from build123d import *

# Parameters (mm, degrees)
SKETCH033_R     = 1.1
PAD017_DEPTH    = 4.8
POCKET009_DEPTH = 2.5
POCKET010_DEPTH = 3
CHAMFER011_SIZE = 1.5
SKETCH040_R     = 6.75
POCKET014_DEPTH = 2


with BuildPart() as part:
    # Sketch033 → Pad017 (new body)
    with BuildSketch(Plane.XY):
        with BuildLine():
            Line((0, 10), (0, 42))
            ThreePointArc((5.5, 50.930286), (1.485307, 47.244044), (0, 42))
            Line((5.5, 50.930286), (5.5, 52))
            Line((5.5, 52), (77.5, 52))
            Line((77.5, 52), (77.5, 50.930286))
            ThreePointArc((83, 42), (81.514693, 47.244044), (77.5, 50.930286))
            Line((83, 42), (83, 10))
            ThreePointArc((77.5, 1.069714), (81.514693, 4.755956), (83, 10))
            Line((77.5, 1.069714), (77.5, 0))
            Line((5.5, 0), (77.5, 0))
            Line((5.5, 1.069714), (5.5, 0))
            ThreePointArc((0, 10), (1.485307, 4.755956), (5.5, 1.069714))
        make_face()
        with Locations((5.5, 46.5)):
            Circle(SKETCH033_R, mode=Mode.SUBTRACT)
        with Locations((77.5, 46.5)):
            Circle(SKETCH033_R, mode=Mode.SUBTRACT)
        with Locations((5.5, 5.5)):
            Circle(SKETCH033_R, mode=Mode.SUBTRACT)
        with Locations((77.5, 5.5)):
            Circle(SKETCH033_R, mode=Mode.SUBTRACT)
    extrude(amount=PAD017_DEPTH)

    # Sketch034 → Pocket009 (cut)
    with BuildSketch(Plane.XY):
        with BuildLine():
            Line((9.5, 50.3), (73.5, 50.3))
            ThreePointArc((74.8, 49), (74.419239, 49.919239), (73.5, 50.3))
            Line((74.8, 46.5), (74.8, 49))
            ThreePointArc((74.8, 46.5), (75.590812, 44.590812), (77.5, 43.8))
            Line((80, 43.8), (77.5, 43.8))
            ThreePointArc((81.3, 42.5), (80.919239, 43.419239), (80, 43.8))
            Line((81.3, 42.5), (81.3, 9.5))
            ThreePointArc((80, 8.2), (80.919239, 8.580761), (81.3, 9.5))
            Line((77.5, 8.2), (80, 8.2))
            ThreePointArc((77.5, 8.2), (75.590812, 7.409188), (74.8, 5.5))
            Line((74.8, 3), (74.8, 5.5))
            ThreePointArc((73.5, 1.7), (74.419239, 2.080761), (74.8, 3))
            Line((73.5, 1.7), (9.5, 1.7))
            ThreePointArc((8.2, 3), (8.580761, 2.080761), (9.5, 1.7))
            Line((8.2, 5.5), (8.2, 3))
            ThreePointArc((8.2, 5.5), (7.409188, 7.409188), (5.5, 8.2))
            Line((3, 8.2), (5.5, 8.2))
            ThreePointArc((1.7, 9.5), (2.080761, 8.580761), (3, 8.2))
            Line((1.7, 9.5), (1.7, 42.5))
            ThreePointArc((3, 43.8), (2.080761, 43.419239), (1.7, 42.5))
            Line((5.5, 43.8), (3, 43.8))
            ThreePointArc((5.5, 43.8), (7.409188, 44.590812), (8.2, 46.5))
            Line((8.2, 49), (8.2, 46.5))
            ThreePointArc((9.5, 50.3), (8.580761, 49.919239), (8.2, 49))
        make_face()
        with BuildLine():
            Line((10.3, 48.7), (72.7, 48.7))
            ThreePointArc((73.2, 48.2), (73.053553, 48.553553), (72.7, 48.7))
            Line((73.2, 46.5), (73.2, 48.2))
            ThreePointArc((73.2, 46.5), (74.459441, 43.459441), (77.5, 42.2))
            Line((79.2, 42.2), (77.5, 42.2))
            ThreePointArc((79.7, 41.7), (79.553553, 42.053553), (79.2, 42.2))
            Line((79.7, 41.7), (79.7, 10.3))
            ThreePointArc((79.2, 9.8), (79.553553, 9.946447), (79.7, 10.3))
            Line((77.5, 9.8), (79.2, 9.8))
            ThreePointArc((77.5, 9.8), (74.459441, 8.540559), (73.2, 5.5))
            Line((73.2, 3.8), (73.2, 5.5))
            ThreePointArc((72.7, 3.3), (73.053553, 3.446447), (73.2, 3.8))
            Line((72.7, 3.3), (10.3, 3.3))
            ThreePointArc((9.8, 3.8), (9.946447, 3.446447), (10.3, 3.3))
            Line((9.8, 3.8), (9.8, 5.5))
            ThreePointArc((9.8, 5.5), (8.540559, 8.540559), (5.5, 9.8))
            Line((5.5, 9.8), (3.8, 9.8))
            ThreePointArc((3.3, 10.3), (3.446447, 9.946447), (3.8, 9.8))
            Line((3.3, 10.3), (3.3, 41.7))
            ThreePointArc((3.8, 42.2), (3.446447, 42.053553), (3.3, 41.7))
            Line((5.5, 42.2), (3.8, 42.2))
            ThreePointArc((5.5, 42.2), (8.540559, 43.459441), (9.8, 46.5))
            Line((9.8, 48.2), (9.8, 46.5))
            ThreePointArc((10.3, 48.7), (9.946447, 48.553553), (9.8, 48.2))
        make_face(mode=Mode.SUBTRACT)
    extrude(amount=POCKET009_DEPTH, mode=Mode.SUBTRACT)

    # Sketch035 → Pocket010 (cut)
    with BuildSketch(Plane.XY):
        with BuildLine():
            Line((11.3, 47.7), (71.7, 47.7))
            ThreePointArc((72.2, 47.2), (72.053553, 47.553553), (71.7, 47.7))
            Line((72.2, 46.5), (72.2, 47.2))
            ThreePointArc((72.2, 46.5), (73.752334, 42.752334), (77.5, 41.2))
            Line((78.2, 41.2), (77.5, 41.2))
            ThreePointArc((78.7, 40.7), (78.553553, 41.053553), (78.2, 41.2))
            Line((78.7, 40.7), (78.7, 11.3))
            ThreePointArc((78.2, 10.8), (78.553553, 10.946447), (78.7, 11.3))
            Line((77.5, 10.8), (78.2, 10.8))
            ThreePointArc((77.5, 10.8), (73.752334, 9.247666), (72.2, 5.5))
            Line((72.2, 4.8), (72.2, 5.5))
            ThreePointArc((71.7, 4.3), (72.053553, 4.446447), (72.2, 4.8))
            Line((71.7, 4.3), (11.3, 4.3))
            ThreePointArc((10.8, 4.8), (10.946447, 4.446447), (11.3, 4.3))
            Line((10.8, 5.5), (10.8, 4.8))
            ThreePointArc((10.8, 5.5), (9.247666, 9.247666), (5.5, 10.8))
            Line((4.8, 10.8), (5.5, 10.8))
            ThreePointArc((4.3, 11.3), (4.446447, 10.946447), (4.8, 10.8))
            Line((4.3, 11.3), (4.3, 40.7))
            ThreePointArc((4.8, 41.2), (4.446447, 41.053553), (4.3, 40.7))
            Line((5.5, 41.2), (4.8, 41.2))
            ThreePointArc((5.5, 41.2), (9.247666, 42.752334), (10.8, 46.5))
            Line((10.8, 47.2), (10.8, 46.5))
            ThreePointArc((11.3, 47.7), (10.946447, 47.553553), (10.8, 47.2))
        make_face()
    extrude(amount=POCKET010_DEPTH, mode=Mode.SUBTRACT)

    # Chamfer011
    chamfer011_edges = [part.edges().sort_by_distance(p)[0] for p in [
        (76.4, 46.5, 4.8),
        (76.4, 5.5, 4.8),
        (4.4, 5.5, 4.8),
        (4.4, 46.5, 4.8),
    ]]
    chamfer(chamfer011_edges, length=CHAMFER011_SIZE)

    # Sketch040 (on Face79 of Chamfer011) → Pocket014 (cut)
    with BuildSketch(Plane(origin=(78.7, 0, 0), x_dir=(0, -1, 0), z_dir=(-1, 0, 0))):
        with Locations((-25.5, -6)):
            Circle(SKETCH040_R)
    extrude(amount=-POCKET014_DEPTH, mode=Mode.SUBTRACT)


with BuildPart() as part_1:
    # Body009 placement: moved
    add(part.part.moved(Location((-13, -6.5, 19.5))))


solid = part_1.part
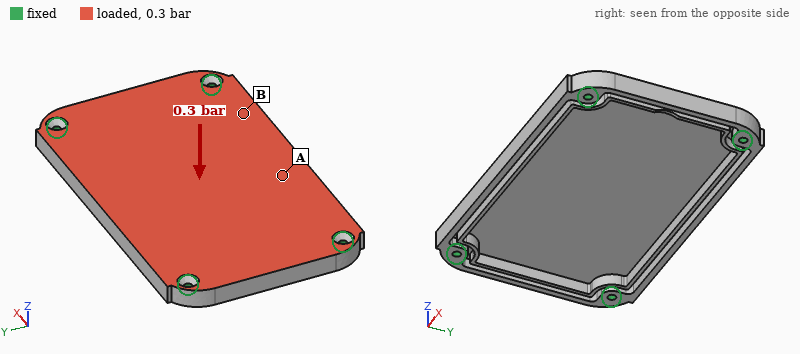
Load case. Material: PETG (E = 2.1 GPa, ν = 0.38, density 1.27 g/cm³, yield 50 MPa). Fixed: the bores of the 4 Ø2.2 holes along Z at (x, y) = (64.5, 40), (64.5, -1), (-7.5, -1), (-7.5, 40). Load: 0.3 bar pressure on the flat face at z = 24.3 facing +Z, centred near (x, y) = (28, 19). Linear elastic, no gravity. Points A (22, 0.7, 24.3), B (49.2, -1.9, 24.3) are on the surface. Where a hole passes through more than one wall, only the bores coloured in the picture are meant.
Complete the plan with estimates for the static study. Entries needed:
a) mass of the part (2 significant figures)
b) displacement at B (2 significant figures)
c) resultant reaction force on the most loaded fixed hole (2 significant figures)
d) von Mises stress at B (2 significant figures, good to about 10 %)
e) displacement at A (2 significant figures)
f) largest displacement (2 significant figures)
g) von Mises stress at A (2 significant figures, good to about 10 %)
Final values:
13 g
0.36 mm
48 N
2.1 MPa
0.75 mm
1.2 mm
5.3 MPa
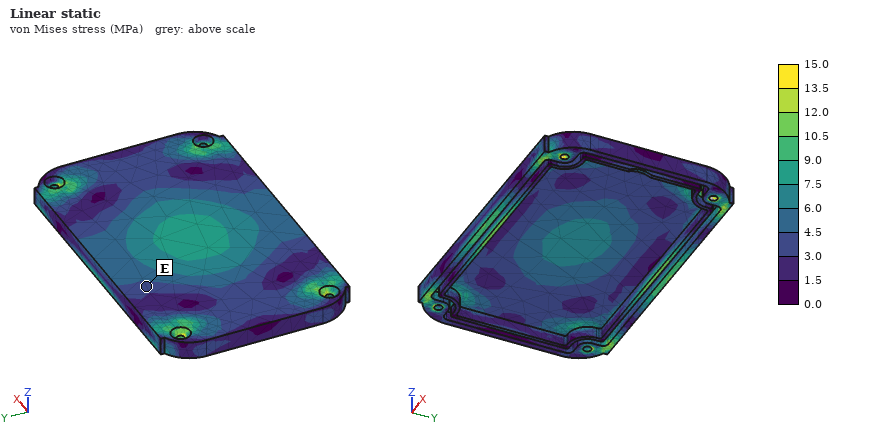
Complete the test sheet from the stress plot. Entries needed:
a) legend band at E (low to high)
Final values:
3.0 to 4.5 MPa
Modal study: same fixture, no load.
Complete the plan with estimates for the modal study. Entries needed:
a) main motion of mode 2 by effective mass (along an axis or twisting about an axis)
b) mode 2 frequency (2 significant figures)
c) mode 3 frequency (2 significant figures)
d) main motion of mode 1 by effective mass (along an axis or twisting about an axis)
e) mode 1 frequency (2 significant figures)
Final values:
twisting about X
960 Hz
1400 Hz
along Z
640 Hz
